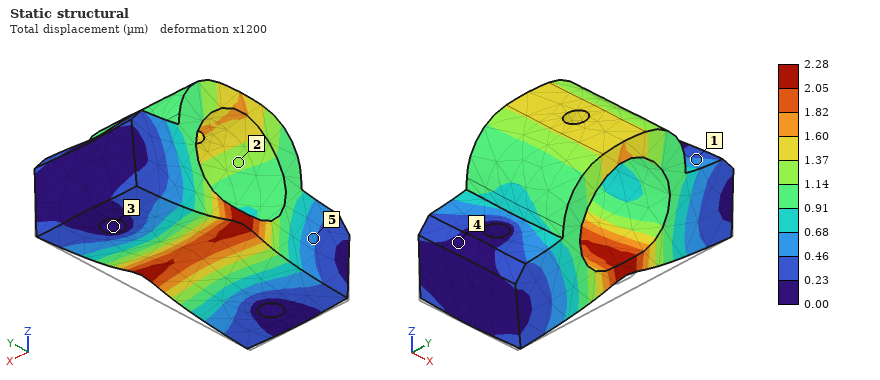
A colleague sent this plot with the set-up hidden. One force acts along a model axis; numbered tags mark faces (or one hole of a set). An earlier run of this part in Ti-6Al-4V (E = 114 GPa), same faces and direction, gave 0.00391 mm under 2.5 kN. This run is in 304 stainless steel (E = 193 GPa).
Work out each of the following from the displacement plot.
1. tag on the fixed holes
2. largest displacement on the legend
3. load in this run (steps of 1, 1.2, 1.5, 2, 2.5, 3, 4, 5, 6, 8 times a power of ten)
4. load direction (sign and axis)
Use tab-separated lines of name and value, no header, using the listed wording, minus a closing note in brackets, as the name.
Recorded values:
tag on the fixed holes	3
largest displacement on the legend	2.28 µm
load in this run	2.5 kN
load direction	+Z
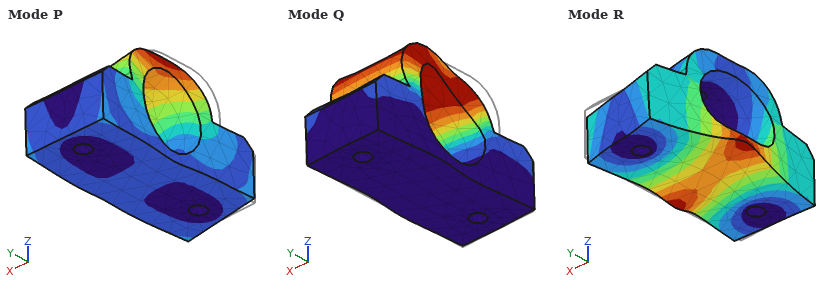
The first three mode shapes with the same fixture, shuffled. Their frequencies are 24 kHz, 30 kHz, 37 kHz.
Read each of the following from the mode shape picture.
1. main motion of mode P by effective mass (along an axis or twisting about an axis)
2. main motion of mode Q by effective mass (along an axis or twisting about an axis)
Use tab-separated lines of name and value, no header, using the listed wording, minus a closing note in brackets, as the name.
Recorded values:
main motion of mode P by effective mass	along X
main motion of mode Q by effective mass	along Y
